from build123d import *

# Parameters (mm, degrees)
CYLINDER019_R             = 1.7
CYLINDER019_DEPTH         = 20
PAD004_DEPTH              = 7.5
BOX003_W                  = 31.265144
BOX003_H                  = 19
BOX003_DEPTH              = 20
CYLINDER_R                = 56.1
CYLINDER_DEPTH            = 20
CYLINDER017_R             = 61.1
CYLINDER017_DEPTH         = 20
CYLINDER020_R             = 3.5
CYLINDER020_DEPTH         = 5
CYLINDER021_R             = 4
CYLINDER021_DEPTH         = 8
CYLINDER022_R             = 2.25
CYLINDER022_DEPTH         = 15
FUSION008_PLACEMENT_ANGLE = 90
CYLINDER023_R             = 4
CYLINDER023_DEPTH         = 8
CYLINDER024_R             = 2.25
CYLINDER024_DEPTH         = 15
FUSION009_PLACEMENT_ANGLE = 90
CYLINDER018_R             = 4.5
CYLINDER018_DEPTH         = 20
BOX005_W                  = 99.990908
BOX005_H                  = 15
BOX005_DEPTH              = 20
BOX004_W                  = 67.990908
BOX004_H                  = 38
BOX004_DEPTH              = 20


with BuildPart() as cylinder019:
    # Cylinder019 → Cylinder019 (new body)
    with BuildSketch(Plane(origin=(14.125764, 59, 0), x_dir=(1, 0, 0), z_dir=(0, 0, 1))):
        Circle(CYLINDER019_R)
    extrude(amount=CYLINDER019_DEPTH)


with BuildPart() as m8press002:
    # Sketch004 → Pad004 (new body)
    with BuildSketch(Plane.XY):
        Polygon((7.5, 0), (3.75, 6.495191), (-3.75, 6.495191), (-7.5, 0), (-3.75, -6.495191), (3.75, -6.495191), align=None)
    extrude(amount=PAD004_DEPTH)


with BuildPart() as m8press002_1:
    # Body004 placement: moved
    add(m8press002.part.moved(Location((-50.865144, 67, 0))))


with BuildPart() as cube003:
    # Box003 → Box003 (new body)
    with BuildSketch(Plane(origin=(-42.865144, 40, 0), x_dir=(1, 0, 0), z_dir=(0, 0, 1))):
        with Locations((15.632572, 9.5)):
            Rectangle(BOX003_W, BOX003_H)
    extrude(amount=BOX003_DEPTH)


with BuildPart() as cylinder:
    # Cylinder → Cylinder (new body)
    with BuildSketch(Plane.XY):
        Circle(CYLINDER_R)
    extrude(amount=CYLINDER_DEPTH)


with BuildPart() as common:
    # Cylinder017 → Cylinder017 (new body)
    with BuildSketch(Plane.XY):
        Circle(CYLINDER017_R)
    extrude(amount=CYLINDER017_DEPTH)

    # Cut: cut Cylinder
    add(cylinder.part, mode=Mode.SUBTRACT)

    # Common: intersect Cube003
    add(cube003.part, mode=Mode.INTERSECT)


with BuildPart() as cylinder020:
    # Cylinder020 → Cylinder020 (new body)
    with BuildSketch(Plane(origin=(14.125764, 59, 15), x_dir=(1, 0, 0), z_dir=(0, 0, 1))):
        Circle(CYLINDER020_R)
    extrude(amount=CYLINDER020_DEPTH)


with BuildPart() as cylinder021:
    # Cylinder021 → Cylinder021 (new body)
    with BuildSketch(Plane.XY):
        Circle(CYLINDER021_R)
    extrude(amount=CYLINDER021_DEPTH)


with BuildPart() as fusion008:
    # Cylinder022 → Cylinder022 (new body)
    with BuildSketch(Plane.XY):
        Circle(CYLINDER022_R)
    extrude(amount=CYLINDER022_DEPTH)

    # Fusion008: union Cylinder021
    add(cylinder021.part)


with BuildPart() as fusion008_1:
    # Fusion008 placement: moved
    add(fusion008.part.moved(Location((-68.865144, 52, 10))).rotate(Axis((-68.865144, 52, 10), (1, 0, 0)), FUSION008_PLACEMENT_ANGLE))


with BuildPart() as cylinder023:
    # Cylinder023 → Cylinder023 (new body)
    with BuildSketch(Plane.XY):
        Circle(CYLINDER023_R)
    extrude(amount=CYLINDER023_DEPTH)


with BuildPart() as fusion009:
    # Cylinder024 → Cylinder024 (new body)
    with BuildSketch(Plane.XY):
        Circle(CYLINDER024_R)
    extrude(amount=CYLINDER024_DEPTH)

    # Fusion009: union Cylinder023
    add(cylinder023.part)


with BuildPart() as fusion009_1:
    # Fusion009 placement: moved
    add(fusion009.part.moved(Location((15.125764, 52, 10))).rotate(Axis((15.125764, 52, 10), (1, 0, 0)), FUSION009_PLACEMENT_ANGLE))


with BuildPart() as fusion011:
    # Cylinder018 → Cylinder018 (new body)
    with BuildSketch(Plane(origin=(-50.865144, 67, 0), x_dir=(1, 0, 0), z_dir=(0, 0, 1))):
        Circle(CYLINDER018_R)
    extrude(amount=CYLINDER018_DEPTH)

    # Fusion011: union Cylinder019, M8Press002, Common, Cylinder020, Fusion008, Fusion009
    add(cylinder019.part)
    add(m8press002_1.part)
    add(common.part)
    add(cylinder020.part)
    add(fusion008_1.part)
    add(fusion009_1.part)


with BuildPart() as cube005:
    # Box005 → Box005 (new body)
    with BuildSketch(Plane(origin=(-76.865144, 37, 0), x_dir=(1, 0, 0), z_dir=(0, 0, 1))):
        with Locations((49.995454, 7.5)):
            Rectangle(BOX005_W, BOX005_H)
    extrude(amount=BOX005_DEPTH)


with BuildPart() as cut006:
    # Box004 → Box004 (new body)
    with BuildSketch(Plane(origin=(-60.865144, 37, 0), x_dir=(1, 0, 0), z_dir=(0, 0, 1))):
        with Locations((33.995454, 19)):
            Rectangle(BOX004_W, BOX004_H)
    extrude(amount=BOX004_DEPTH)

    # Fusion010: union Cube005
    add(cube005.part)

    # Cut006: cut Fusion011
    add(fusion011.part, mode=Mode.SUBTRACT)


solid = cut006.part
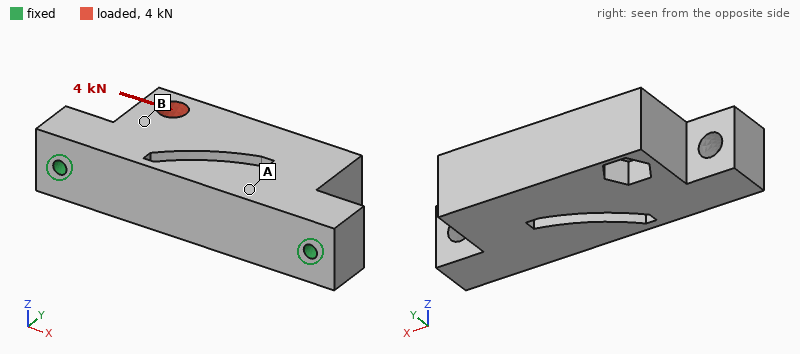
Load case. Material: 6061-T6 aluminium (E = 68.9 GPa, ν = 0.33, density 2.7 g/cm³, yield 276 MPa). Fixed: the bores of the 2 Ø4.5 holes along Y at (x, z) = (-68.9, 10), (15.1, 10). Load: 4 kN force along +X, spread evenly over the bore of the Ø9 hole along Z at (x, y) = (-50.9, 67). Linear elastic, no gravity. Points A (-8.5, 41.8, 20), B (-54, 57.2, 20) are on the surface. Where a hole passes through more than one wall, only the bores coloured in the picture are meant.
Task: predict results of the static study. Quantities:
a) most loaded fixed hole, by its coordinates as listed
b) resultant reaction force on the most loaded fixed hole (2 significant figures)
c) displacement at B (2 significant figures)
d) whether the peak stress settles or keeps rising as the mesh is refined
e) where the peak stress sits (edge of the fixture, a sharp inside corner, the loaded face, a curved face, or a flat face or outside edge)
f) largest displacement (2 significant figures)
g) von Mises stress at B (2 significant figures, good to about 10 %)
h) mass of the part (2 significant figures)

(-68.9, 10)
2.6 kN
11 µm
keeps rising
edge of the fixture
19 µm
12 MPa
150 g
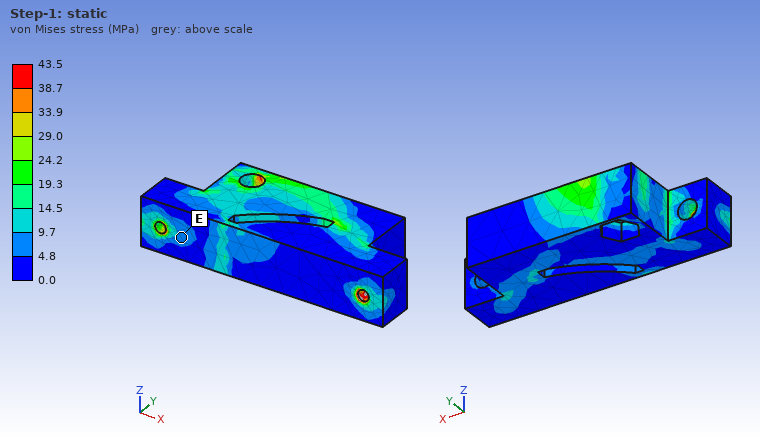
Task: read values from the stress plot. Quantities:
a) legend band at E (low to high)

4.8 to 9.7 MPa
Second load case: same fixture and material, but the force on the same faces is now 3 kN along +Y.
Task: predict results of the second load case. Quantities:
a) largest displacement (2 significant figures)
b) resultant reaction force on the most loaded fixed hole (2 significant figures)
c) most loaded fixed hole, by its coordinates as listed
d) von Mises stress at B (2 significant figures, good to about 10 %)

35 µm
2.5 kN
(-68.9, 10)
16 MPa
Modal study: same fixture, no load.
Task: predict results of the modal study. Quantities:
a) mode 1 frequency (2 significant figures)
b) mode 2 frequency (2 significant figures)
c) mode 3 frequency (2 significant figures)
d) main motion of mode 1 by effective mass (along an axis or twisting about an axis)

2900 Hz
8300 Hz
8400 Hz
along Z
